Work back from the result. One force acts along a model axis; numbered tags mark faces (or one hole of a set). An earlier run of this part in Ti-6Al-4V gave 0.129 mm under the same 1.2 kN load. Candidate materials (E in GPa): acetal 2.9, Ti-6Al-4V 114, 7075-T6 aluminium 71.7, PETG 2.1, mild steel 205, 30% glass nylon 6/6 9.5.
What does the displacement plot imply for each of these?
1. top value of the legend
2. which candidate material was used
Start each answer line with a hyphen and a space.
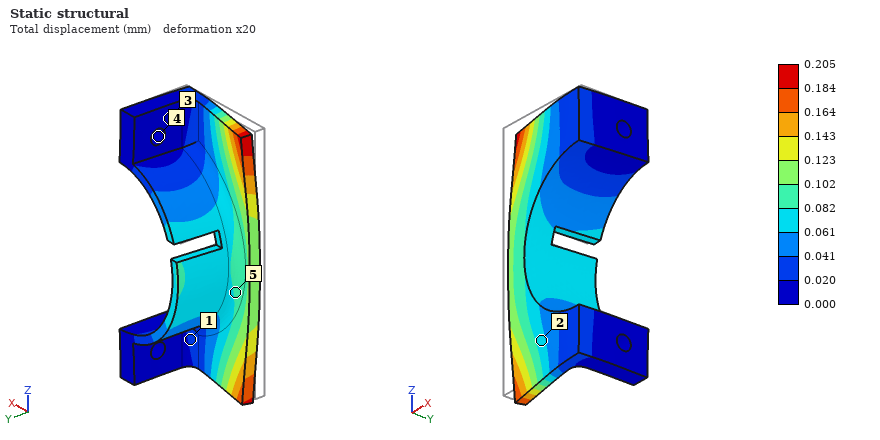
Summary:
- 0.205 mm
- 7075-T6 aluminium
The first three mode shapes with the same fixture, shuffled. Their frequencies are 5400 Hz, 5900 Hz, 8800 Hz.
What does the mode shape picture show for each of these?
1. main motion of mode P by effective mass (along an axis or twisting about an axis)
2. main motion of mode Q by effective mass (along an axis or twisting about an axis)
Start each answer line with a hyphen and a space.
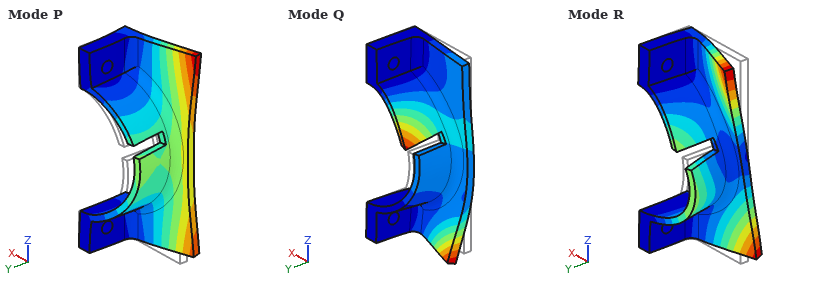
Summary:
- along Y
- along Z
